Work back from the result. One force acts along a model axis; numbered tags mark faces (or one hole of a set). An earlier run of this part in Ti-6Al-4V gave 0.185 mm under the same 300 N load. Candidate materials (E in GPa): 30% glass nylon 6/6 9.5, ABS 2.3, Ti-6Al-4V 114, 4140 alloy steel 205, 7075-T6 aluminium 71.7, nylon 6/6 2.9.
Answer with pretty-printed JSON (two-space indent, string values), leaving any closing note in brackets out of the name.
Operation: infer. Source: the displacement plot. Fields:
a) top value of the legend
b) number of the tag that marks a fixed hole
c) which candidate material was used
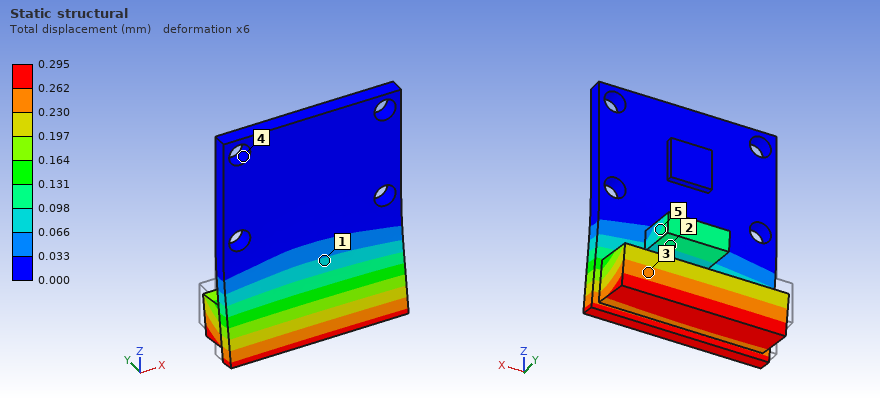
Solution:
{
  "top value of the legend": "0.295 mm",
  "number of the tag that marks a fixed hole": "4",
  "which candidate material was used": "7075-T6 aluminium"
}
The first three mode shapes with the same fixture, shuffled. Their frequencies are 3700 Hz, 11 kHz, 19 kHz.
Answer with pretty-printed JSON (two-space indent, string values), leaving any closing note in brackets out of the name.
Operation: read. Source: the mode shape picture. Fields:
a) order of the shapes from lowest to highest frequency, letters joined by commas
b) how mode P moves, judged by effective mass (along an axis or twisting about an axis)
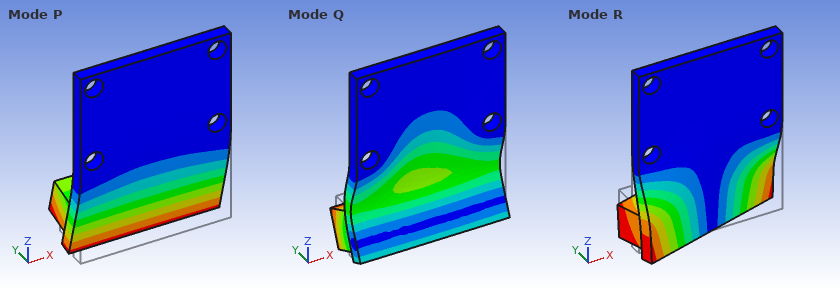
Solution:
{
  "order of the shapes from lowest to highest frequency, letters joined by commas": "P, R, Q",
  "how mode P moves, judged by effective mass": "along Y"
}
